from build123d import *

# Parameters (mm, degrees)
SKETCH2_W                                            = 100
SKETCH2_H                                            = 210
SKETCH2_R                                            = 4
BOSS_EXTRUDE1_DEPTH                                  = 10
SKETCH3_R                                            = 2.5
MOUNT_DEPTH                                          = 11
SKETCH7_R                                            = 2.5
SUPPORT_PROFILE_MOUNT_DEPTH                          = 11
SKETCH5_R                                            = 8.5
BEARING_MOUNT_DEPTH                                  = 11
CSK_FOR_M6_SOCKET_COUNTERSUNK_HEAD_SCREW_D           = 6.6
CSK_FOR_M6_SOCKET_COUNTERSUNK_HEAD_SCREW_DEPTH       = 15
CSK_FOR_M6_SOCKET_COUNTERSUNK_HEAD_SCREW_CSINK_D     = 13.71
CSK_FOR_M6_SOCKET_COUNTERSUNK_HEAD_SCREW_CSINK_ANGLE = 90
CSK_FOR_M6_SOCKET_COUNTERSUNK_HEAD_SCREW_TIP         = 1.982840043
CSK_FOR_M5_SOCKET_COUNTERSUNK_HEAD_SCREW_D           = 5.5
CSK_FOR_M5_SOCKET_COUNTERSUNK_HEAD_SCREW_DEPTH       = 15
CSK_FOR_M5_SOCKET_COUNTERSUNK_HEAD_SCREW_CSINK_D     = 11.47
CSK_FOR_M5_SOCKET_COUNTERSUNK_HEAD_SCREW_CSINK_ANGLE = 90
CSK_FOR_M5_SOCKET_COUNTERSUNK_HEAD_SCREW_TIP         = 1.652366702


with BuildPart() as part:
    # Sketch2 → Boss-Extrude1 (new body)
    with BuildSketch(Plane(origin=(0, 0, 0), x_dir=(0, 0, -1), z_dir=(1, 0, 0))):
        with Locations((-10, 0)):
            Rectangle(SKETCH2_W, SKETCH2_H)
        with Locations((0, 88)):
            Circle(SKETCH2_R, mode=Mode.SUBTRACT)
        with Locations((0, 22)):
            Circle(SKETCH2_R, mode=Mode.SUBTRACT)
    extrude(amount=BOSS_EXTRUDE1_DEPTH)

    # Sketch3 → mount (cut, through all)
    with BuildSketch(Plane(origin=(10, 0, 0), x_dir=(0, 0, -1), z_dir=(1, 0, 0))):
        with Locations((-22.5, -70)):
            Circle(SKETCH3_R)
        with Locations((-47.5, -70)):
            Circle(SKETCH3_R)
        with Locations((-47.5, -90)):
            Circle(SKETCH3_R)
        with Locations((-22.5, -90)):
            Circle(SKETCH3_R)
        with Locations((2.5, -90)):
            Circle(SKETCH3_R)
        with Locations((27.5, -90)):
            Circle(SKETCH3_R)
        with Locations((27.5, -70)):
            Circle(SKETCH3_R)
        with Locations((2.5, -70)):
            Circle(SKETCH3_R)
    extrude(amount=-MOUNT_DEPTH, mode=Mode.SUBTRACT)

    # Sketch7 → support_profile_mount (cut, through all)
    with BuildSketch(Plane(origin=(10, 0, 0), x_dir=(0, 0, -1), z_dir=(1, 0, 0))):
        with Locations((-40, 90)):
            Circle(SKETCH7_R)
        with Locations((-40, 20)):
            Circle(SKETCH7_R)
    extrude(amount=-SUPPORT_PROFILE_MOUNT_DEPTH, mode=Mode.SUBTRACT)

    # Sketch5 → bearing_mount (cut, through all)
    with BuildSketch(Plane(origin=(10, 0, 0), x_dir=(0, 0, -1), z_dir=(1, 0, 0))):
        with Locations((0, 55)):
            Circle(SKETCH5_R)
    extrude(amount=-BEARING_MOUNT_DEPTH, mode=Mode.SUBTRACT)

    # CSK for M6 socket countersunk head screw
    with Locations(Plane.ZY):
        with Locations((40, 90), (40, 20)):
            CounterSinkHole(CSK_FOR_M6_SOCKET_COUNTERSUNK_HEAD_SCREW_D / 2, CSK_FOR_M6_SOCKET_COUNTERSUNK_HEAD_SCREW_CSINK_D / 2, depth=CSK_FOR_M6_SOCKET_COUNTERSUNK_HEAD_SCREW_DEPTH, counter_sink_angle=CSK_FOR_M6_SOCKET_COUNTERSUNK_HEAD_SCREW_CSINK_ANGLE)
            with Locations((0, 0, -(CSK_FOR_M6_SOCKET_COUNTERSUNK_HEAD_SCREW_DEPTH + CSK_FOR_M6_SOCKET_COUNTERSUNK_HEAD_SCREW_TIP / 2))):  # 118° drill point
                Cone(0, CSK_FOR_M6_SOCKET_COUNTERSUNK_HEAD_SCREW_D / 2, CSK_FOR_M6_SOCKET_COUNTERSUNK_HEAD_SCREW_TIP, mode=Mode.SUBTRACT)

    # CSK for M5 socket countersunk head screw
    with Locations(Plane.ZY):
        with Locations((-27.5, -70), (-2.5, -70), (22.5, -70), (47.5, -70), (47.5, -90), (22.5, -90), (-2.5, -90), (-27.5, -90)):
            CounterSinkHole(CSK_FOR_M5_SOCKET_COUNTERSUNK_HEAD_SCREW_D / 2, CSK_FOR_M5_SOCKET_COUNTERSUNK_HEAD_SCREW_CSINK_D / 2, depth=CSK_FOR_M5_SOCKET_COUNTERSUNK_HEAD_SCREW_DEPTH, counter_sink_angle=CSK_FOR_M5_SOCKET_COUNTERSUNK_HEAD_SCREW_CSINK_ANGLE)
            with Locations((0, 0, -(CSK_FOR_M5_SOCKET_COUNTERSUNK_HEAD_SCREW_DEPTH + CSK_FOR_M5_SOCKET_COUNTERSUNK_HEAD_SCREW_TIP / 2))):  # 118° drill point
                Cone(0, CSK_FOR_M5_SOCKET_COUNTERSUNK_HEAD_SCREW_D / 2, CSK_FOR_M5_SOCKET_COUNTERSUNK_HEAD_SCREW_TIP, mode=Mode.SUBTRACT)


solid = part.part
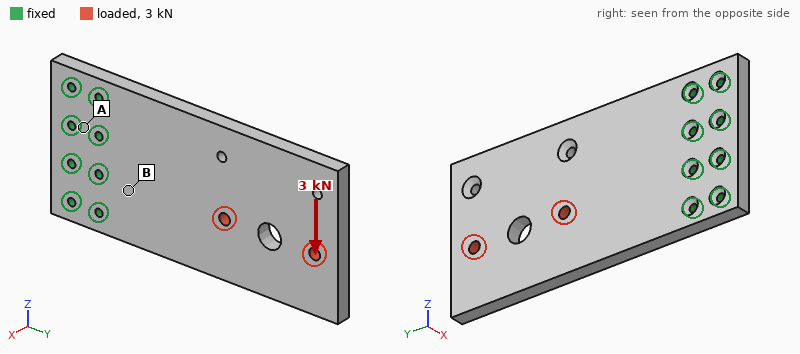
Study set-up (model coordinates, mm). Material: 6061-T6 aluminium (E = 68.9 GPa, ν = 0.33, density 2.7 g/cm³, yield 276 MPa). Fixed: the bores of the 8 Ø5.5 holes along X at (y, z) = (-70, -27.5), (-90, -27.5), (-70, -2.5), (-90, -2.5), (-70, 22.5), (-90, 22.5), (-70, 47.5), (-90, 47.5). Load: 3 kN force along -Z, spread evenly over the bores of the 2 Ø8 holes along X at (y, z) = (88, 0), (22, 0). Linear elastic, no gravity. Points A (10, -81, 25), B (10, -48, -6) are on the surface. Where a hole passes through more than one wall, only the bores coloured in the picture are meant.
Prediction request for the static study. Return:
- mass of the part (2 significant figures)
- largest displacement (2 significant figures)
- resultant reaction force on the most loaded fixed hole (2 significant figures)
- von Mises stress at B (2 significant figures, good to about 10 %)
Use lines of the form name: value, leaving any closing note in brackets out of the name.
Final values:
mass of the part: 550 g
largest displacement: 86 µm
resultant reaction force on the most loaded fixed hole: 3.6 kN
von Mises stress at B: 9.6 MPa
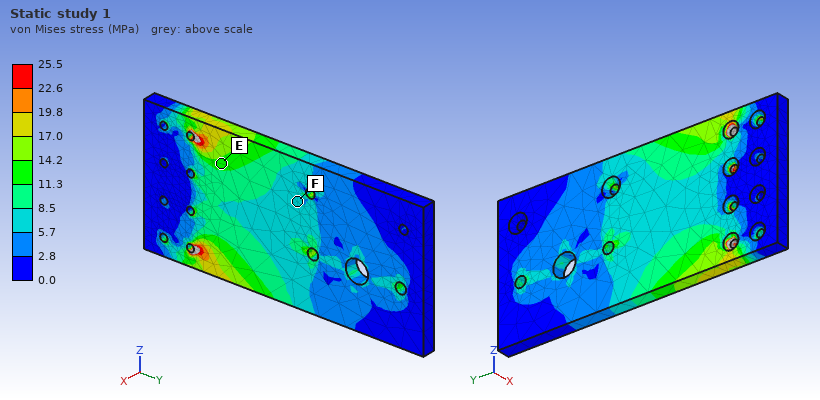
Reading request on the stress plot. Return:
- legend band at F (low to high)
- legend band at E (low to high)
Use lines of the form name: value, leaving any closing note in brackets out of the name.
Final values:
legend band at F: 5.7 to 8.5 MPa
legend band at E: 11.3 to 14.2 MPa
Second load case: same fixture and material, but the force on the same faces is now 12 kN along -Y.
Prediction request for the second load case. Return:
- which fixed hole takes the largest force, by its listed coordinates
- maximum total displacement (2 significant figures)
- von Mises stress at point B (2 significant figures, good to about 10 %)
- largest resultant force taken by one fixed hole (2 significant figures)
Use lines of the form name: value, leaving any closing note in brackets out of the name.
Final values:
which fixed hole takes the largest force, by its listed coordinates: (-70, -27.5)
maximum total displacement: 52 µm
von Mises stress at point B: 15 MPa
largest resultant force taken by one fixed hole: 3.7 kN
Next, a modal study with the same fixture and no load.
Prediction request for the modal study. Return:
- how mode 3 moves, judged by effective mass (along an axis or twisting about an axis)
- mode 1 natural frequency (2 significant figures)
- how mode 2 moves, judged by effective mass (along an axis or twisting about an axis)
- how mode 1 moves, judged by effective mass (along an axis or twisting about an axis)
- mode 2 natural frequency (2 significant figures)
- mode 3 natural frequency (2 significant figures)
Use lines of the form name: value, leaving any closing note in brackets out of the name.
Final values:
how mode 3 moves, judged by effective mass: along X
mode 1 natural frequency: 270 Hz
how mode 2 moves, judged by effective mass: twisting about Y
how mode 1 moves, judged by effective mass: along X
mode 2 natural frequency: 970 Hz
mode 3 natural frequency: 1600 Hz
